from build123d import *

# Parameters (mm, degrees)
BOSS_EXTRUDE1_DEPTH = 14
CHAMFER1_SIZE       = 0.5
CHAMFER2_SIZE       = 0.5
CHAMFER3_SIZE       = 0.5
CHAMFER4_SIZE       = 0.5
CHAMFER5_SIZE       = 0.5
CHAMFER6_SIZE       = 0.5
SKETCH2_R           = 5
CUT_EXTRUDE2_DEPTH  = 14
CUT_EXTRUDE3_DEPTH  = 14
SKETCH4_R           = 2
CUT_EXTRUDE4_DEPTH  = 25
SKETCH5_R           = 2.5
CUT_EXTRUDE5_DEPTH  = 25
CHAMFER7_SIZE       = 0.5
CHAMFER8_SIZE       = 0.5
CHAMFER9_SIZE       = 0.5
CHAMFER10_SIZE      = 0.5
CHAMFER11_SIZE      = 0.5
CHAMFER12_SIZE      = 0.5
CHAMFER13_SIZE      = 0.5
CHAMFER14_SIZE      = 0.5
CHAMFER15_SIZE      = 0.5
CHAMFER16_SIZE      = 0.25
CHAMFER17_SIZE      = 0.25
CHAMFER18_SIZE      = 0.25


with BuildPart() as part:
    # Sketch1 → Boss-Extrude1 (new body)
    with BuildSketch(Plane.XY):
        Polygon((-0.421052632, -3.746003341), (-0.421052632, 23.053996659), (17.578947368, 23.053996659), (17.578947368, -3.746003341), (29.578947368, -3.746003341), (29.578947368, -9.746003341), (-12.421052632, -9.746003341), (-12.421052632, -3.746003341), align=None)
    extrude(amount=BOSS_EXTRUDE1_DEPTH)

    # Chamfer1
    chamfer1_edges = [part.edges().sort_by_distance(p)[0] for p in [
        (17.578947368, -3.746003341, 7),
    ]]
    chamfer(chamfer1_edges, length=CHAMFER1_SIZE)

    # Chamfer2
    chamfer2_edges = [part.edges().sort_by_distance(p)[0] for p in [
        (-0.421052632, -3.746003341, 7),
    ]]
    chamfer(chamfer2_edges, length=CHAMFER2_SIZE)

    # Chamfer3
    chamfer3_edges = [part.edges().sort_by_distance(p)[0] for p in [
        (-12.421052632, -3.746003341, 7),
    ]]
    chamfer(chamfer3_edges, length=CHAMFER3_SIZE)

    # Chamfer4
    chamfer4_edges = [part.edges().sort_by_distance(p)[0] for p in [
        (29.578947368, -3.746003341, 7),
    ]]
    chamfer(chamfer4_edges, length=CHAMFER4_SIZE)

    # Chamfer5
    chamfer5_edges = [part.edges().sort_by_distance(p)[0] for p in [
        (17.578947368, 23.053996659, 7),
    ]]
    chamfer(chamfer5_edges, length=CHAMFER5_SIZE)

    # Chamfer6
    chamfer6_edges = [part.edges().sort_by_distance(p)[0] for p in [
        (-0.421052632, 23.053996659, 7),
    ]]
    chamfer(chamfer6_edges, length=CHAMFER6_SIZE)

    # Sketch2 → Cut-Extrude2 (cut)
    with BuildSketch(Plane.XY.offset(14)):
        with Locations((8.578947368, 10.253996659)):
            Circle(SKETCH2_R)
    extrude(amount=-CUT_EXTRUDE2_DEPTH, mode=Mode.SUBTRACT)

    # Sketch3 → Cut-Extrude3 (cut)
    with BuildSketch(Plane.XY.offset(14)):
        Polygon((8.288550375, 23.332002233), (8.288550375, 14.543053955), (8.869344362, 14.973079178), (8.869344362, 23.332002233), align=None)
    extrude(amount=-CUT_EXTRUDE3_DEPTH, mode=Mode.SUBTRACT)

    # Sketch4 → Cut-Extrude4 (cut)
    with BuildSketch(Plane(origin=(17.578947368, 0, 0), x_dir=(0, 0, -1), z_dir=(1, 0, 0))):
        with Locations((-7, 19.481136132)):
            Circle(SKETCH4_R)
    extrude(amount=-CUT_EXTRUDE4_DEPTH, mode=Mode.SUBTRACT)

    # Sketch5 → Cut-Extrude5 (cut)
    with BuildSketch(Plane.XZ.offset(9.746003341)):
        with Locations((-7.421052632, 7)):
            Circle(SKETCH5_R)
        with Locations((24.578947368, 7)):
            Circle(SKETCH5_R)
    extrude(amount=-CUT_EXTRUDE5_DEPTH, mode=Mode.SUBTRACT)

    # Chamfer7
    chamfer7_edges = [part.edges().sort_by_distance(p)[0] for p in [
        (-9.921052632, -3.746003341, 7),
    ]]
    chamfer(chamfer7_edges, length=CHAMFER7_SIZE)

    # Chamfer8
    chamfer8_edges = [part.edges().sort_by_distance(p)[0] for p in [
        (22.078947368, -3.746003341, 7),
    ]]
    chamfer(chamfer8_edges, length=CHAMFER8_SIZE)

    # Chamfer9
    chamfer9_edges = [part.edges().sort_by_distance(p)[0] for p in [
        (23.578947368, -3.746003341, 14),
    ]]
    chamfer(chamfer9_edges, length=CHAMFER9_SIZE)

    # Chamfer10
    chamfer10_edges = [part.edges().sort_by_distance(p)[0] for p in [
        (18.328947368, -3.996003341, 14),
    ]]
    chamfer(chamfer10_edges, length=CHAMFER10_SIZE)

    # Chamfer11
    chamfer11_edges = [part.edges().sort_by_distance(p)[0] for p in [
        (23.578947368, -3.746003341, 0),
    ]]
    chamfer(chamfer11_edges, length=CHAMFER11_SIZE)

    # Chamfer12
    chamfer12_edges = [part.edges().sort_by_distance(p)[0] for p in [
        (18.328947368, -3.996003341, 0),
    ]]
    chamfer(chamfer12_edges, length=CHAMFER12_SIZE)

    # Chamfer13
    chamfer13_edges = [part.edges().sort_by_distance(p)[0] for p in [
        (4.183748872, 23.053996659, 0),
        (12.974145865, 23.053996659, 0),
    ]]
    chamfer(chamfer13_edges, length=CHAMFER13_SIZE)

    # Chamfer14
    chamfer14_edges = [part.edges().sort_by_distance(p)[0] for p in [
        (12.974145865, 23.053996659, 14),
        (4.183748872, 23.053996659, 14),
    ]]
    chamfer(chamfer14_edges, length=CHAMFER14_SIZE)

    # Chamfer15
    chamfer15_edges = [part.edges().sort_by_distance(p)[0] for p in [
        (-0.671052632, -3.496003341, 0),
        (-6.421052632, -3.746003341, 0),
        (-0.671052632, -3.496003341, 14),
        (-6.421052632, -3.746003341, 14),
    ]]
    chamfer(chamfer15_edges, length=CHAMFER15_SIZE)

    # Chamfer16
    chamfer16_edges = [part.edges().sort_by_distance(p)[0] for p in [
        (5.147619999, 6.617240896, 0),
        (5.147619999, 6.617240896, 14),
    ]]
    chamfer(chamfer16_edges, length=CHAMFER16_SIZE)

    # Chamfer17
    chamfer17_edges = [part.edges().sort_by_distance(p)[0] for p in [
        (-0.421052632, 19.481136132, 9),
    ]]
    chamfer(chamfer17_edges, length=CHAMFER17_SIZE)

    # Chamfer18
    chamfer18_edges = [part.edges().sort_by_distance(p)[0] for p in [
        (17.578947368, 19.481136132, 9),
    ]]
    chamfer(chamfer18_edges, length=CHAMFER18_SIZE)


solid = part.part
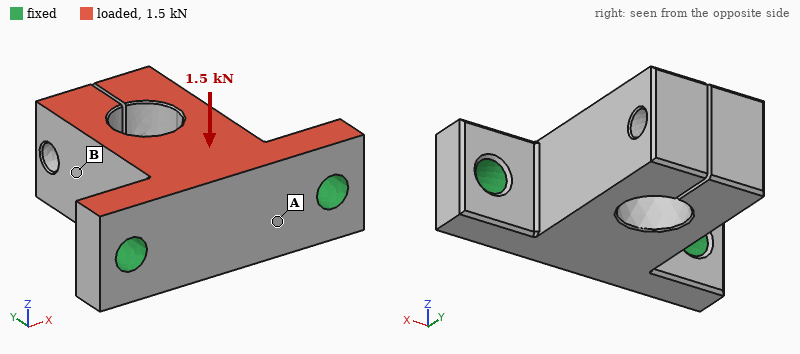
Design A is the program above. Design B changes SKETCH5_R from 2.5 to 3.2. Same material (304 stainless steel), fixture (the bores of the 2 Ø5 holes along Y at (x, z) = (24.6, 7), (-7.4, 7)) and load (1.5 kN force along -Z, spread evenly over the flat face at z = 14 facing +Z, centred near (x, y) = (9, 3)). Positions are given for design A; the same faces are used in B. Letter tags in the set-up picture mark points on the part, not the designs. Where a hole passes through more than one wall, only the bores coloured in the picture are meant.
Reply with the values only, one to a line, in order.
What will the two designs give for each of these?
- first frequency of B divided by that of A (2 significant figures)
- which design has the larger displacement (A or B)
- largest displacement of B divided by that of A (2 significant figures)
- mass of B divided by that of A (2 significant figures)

1.1
A
0.86
0.98
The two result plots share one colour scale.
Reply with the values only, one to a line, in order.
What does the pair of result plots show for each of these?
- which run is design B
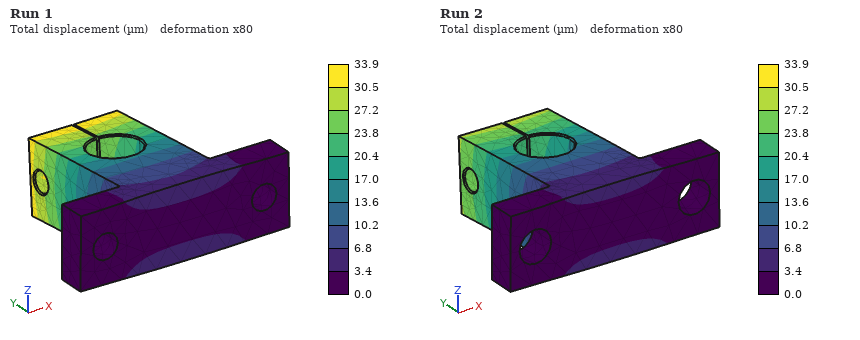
Run 2
